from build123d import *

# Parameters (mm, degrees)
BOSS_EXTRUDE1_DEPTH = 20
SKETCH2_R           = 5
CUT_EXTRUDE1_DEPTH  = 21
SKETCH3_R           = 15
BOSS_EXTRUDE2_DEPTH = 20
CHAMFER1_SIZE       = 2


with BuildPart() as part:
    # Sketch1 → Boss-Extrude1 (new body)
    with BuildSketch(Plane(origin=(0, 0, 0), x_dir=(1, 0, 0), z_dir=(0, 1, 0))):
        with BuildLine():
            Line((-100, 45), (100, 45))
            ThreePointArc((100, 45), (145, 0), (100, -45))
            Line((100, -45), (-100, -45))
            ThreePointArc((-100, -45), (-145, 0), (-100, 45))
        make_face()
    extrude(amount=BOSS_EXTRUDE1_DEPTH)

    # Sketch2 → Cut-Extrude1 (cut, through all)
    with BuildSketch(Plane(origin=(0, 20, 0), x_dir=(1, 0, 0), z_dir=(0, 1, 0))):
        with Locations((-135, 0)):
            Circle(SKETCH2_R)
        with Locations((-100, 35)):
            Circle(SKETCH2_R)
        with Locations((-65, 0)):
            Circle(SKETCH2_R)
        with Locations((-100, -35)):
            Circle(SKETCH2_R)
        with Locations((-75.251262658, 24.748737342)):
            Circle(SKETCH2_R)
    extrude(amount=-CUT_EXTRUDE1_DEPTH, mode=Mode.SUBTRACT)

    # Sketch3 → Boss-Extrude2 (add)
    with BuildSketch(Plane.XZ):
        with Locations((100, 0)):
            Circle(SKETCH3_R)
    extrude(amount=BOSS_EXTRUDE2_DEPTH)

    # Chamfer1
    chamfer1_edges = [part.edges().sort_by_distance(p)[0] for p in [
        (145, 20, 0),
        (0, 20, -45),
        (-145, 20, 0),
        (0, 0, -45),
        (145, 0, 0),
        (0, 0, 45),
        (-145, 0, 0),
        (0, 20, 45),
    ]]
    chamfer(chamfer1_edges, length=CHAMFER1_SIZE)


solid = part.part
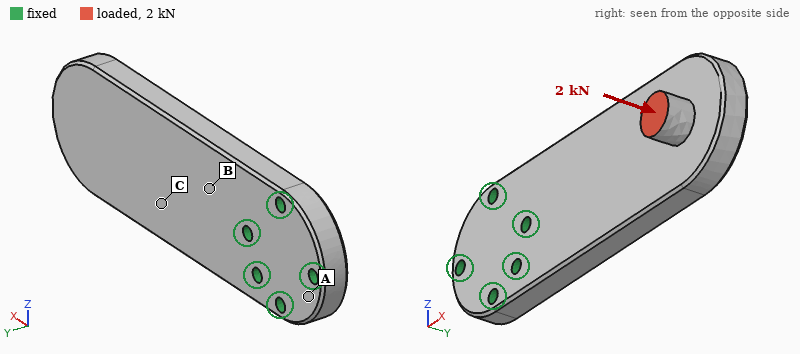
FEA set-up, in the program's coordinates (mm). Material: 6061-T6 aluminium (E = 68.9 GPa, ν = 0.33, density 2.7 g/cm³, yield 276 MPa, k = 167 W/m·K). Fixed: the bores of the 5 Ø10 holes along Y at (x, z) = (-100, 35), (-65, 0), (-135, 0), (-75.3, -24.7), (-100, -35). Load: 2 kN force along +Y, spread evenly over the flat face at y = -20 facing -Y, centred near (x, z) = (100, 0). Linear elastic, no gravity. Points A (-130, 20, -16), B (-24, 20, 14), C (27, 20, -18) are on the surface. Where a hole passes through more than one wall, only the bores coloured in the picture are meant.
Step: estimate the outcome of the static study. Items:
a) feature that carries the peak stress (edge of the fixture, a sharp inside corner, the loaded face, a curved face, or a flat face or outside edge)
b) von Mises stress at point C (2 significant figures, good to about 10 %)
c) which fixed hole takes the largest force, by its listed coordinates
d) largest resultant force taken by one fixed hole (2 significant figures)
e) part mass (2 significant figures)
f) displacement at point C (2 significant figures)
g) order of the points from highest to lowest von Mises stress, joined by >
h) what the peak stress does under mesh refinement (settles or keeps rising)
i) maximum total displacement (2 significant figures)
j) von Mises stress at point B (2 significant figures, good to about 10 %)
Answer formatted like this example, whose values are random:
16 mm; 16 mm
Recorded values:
edge of the fixture; 24 MPa; (-65, 0); 5.9 kN; 1.3 kg; 0.31 mm; B > C > A; keeps rising; 1.1 mm; 39 MPa
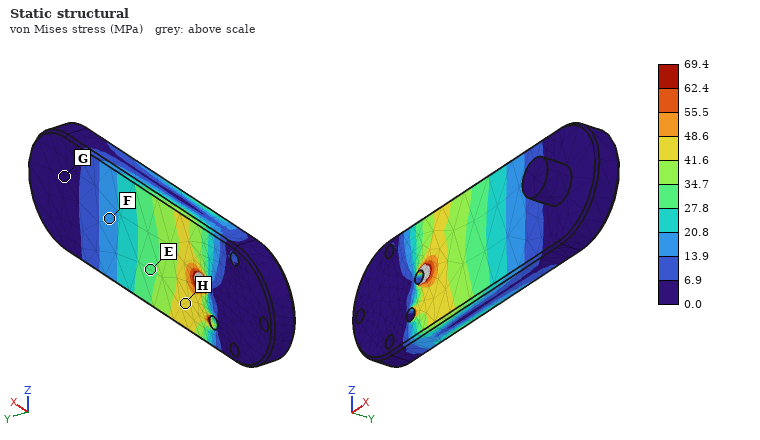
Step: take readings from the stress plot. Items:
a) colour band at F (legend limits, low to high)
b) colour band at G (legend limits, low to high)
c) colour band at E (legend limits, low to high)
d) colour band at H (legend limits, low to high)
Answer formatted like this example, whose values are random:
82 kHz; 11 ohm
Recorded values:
13.9 to 20.8 MPa; 0.0 to 6.9 MPa; 27.8 to 34.7 MPa; 41.6 to 48.6 MPa
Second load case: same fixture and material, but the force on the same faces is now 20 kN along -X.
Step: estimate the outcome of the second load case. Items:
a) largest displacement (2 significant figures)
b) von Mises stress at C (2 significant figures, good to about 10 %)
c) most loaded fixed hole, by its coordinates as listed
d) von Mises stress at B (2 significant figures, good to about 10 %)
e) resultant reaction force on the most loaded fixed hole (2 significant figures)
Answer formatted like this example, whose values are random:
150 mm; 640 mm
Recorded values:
3.1 mm; 87 MPa; (-65, 0); 84 MPa; 13 kN
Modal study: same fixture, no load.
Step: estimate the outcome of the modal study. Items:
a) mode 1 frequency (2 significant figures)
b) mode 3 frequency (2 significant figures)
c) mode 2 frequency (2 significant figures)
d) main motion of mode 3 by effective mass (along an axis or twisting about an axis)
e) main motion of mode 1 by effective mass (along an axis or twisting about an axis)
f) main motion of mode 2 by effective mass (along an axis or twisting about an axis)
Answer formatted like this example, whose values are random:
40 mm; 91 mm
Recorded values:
370 Hz; 1600 Hz; 1300 Hz; twisting about X; along Y; along Z
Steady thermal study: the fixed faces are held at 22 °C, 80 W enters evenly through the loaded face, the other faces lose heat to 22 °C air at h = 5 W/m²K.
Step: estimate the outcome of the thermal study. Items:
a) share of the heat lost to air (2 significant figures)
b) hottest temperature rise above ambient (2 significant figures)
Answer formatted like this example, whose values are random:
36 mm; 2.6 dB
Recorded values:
7.8 %; 60 K
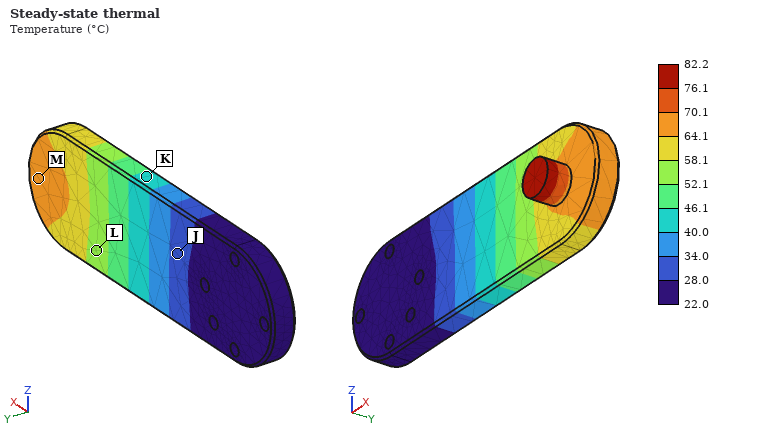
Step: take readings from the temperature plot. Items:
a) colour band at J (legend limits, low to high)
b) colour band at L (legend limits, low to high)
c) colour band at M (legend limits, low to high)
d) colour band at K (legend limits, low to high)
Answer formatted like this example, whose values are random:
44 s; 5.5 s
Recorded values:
28.0 to 34.0 °C; 52.1 to 58.1 °C; 64.1 to 70.1 °C; 40.0 to 46.1 °C
